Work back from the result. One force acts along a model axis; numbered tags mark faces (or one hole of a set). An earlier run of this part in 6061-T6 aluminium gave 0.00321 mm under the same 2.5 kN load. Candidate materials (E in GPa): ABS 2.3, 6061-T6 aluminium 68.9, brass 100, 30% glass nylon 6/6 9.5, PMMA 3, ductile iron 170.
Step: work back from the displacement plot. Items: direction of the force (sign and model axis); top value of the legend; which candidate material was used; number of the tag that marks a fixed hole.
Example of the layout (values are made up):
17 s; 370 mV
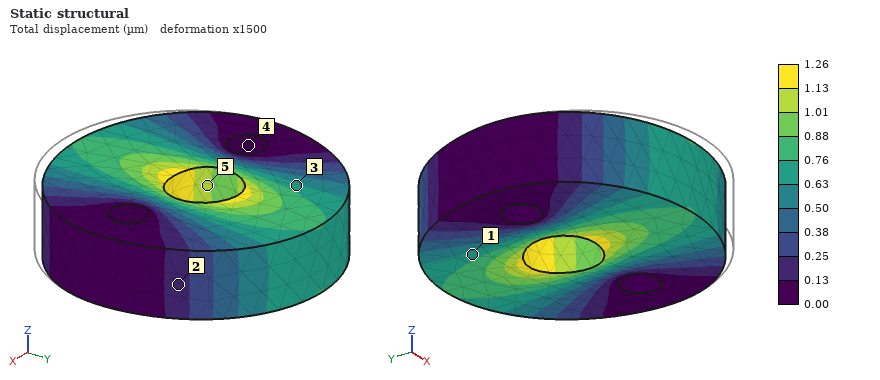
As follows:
+Y; 1.26 µm; ductile iron; 4
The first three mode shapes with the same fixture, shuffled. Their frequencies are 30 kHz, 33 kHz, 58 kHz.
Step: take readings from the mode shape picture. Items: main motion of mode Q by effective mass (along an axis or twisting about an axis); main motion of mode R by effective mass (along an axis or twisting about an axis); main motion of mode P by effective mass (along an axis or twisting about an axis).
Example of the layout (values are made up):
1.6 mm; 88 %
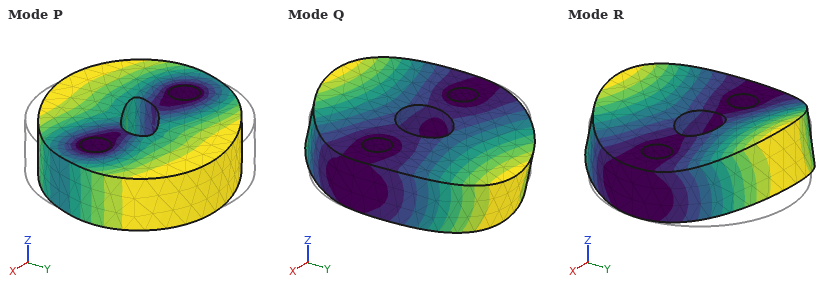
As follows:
twisting about X; along Z; twisting about Z
